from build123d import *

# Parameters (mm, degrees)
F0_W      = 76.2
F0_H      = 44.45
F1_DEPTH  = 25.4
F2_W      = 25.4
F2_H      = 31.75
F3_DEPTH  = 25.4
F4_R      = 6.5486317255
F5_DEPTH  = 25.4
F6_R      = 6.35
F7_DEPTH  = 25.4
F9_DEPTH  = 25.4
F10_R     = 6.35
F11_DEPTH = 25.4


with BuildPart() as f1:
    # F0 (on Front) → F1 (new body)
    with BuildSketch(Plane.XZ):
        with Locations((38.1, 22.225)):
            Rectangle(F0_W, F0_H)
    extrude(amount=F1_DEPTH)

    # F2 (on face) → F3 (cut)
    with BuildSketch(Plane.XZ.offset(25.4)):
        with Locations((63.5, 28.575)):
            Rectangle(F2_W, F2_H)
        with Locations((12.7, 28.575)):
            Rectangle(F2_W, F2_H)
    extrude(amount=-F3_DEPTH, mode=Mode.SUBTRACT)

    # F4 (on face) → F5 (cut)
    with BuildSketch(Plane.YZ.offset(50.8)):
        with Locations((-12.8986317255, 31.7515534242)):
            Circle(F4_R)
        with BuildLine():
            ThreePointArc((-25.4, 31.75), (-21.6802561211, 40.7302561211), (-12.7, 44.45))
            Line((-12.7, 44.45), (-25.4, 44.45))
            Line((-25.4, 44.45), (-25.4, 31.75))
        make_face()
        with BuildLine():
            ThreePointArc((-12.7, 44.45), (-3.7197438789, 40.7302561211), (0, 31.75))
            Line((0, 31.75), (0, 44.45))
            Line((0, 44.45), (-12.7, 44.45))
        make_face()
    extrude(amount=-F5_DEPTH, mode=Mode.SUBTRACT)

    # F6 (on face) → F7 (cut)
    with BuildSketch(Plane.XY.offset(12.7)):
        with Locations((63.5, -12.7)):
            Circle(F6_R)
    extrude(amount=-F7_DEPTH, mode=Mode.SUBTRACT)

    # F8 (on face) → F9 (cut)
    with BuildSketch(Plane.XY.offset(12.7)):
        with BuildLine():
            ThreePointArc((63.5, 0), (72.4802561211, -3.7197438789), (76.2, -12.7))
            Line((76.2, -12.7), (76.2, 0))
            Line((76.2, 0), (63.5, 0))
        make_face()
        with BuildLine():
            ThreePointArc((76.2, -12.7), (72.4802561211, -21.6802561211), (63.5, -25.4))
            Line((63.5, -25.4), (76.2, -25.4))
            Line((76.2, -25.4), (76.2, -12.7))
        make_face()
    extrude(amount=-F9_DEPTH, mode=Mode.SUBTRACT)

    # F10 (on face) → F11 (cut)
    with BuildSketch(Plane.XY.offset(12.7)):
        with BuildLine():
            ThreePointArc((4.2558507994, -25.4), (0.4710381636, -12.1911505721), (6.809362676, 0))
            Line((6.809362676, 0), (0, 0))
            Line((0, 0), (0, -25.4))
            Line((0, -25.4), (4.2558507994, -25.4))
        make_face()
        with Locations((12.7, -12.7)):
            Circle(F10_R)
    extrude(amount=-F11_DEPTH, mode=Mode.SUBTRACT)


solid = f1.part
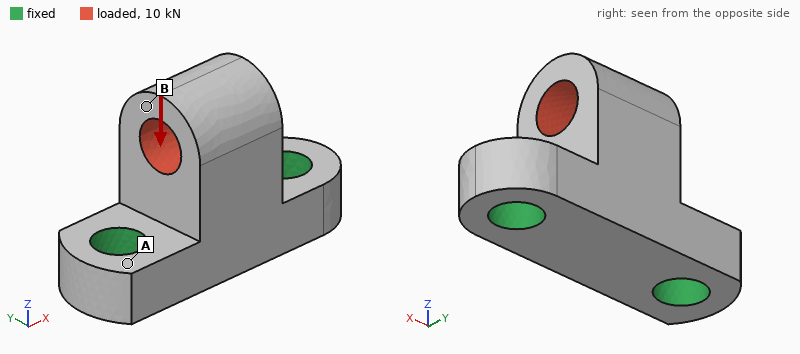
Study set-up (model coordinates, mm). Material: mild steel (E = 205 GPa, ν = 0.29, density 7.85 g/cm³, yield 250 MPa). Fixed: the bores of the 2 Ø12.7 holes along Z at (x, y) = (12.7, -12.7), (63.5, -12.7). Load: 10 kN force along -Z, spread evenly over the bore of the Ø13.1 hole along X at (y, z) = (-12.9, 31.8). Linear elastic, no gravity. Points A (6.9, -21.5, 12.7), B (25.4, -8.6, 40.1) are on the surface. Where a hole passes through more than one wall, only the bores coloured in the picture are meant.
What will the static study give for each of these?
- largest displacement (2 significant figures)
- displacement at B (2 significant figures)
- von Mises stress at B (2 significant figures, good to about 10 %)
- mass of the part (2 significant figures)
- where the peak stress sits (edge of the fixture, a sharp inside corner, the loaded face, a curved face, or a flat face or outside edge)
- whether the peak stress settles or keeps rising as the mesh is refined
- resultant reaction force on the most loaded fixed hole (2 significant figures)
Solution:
7.9 µm
7.2 µm
16 MPa
280 g
edge of the fixture
keeps rising
5.2 kN
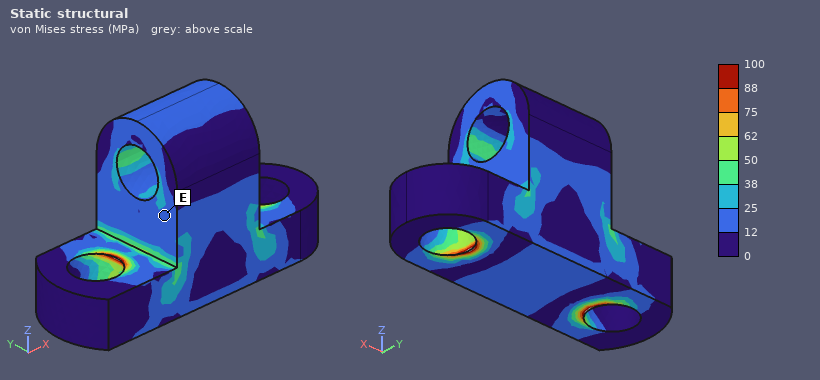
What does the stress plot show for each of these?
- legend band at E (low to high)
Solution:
12 to 25 MPa
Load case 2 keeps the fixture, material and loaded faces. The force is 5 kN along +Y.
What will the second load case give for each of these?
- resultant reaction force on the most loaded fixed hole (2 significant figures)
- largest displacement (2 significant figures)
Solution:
2.5 kN
37 µm
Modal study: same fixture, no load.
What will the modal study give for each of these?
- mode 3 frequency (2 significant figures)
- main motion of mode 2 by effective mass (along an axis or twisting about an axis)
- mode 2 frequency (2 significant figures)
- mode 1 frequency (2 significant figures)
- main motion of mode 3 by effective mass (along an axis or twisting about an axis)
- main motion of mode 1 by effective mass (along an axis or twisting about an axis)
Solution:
17 kHz
along X
12 kHz
7100 Hz
along Z
along Y
